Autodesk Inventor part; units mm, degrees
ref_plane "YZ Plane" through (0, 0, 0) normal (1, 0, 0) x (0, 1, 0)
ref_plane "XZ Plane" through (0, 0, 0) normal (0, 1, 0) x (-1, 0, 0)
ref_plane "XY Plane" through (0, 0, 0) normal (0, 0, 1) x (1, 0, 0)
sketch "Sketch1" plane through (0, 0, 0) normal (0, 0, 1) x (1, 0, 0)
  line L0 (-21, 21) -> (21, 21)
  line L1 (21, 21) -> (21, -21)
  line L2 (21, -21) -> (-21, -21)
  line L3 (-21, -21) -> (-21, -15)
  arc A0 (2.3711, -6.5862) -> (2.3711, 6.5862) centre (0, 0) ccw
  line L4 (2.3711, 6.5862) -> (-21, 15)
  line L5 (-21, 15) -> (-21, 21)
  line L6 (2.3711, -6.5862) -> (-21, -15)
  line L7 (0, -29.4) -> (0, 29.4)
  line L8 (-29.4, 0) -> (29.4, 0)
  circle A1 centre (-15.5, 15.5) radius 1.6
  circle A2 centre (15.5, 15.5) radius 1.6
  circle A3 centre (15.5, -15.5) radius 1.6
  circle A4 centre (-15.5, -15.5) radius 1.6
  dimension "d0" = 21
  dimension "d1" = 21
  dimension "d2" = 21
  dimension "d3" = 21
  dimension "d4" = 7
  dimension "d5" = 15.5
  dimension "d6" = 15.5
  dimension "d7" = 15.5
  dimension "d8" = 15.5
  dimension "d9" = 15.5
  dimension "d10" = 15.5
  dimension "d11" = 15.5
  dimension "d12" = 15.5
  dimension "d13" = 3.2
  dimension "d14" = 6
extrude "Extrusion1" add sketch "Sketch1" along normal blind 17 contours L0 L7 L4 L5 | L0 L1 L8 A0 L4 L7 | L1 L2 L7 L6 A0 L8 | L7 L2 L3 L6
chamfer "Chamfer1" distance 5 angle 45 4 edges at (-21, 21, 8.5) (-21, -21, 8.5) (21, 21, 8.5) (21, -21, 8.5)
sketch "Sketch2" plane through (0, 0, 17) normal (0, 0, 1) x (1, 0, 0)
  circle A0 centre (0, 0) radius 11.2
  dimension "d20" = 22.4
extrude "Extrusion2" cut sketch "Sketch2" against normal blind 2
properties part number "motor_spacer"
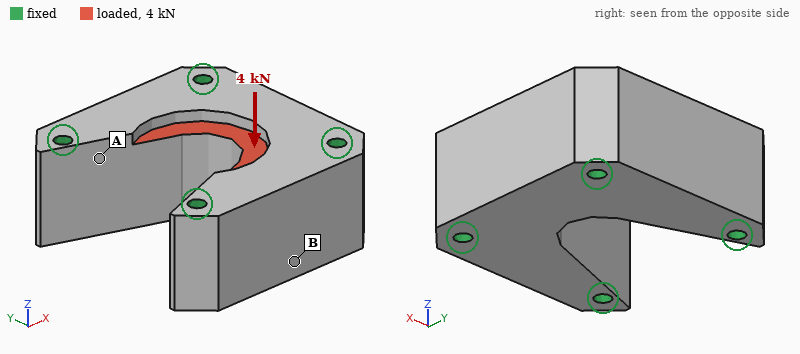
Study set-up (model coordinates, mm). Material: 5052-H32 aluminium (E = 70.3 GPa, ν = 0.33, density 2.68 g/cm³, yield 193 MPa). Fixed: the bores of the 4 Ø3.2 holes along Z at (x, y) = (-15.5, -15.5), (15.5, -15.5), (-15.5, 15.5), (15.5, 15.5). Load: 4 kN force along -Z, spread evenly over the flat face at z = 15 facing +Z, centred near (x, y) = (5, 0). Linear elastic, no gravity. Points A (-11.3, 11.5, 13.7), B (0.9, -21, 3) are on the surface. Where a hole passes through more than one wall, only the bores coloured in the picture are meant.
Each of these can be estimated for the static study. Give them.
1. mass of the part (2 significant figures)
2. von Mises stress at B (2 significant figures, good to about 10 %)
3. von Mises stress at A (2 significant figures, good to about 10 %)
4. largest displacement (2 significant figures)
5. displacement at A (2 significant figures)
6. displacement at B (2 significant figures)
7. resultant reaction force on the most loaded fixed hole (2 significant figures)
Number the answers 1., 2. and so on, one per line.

1. 51 g
2. 5.4 MPa
3. 14 MPa
4. 8.0 µm
5. 1.5 µm
6. 1.7 µm
7. 1.4 kN
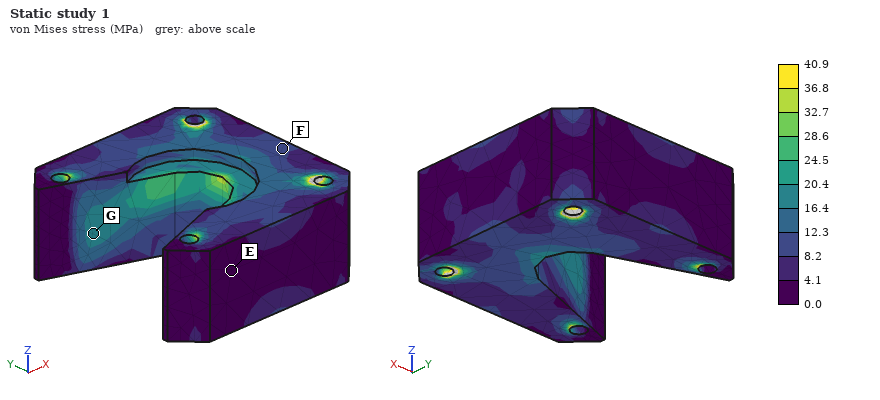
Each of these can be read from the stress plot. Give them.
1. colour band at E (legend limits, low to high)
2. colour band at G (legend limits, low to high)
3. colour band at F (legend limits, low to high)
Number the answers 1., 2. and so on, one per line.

1. 0.0 to 4.1 MPa
2. 16.4 to 20.4 MPa
3. 8.2 to 12.3 MPa
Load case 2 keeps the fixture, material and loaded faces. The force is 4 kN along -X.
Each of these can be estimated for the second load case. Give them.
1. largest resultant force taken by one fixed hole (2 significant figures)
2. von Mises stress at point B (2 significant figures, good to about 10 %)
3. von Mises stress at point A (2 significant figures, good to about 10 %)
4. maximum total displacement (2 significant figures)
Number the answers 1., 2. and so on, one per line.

1. 1.4 kN
2. 4.7 MPa
3. 12 MPa
4. 8.5 µm
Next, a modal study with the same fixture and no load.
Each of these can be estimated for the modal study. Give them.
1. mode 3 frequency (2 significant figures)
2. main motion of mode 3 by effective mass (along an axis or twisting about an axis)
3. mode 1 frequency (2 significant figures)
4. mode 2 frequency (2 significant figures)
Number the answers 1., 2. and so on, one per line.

1. 38 kHz
2. along Y
3. 33 kHz
4. 34 kHz
